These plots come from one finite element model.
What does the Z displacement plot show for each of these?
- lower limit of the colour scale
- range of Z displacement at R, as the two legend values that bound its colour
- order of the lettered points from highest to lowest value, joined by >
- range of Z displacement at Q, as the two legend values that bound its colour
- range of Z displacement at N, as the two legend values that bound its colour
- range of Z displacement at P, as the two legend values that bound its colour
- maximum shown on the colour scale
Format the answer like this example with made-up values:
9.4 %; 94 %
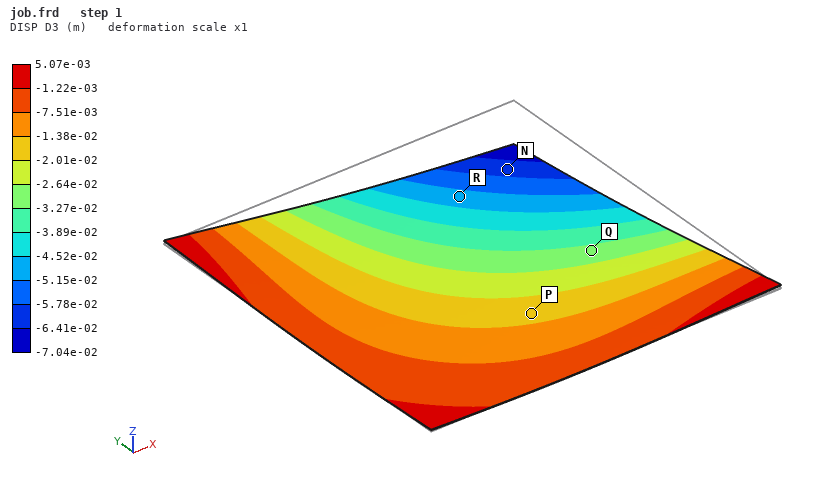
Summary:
-7.04e-02 m; -5.15e-02 to -4.52e-02 m; P > Q > R > N; -3.27e-02 to -2.64e-02 m; -6.41e-02 to -5.78e-02 m; -2.01e-02 to -1.38e-02 m; 5.07e-03 m
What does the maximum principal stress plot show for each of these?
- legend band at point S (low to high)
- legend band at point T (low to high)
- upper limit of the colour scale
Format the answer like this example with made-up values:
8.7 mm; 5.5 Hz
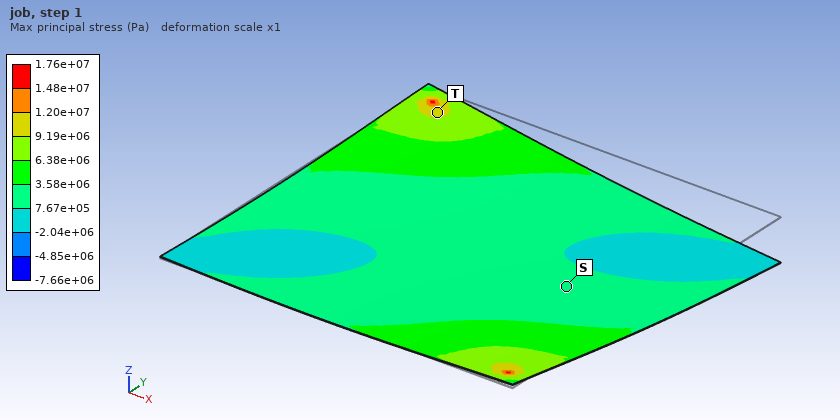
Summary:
7.67e+05 to 3.58e+06 Pa; 9.19e+06 to 1.20e+07 Pa; 1.76e+07 Pa
